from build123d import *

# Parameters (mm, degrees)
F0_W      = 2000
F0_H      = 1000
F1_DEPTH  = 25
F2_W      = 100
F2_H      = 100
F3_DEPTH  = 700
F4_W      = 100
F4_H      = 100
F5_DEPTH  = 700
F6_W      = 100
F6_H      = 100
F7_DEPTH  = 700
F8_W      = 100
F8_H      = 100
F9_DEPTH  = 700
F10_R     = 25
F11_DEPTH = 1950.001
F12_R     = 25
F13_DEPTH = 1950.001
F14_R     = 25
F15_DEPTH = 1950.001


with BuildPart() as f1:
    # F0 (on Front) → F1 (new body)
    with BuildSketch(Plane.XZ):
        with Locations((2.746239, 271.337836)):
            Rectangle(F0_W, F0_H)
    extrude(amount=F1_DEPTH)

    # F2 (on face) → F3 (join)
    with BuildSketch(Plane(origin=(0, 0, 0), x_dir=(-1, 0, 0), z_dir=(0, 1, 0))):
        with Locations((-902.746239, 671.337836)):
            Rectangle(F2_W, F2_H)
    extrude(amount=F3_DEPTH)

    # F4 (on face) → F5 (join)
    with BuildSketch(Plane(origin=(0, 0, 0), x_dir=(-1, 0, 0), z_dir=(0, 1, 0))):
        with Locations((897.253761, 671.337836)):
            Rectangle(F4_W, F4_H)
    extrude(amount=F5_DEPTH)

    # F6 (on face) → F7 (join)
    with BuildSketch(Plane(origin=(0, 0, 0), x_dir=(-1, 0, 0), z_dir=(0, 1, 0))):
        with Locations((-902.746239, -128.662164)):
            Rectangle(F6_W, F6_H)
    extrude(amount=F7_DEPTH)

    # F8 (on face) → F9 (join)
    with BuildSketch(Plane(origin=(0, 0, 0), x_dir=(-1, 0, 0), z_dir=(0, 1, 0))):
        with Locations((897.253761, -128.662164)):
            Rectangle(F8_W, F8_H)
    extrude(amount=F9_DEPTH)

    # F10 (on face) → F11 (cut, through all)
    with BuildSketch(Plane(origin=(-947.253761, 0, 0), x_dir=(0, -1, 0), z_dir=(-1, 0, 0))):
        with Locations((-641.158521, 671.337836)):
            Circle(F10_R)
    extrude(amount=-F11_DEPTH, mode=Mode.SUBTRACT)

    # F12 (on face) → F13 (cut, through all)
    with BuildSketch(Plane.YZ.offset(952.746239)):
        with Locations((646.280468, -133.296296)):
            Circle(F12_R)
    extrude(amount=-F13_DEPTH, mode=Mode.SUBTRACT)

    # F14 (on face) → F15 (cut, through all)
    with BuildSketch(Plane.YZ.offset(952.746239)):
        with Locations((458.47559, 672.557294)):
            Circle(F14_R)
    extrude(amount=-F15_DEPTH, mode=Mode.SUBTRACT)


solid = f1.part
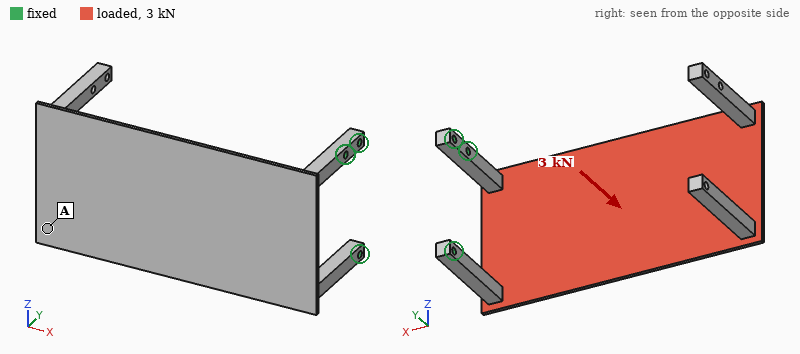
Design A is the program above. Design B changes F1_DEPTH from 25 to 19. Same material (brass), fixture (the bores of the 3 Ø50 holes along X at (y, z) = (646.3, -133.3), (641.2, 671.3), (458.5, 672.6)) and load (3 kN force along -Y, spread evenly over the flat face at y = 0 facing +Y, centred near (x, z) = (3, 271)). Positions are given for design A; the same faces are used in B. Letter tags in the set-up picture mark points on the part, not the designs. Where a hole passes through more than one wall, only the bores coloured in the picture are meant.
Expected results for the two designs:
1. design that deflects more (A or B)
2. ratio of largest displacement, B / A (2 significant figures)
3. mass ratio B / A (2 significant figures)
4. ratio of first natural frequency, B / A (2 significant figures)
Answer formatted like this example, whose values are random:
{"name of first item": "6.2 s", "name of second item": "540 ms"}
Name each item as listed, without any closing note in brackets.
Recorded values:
{"design that deflects more": "B", "ratio of largest displacement, B / A": "2.2", "mass ratio B / A": "0.84", "ratio of first natural frequency, B / A": "0.72"}
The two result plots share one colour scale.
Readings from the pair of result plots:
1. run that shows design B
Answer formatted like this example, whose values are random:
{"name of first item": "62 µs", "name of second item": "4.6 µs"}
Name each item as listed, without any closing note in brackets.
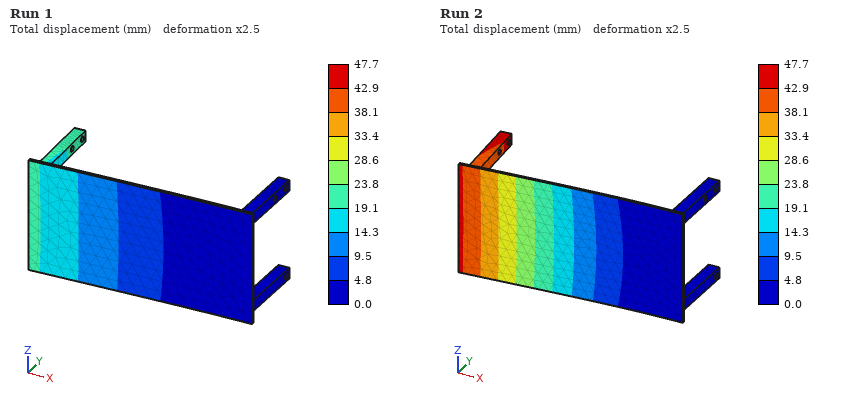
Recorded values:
{"run that shows design B": "Run 2"}
